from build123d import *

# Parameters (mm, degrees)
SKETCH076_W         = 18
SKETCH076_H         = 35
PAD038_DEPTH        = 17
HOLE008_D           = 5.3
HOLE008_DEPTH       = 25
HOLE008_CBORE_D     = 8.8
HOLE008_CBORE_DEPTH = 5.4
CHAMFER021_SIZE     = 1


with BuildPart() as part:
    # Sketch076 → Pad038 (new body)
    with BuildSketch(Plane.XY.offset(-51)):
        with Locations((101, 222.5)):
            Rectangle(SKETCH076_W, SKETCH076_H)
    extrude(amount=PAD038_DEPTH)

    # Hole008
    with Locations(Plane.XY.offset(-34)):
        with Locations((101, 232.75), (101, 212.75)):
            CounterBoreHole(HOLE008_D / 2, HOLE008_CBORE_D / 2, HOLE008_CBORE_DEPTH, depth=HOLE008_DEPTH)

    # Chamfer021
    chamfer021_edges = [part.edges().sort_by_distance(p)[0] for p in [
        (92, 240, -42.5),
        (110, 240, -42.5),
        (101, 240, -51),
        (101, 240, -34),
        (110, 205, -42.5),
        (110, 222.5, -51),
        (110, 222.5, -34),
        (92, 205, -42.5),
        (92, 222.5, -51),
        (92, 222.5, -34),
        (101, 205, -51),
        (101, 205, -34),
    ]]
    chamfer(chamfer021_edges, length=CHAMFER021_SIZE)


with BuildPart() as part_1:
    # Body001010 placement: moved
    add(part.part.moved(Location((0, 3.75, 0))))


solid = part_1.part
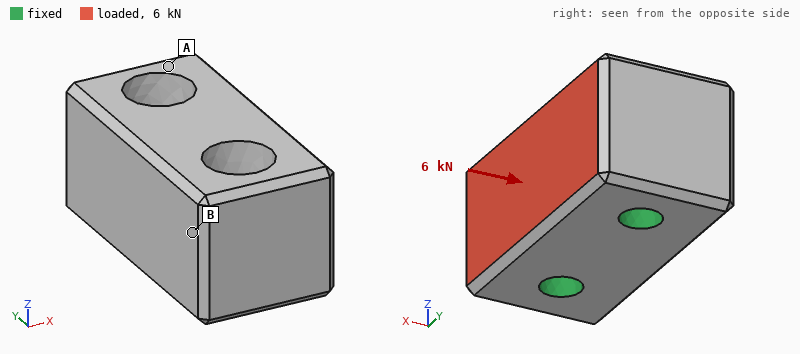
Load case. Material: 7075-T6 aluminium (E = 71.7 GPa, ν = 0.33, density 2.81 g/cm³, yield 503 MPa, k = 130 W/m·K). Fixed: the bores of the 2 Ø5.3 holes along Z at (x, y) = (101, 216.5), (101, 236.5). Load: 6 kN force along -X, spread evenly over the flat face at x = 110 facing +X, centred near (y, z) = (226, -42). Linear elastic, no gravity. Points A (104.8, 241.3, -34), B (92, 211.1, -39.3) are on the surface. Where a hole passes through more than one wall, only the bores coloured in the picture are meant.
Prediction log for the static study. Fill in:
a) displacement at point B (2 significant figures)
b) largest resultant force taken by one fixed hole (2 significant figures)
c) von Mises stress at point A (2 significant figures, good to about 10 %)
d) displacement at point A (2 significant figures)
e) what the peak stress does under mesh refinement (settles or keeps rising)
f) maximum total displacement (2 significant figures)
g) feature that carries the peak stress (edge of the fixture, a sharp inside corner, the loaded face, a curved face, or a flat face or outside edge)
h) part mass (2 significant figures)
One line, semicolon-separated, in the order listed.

1.9 µm; 3.1 kN; 12 MPa; 3.6 µm; keeps rising; 5.3 µm; edge of the fixture; 26 g
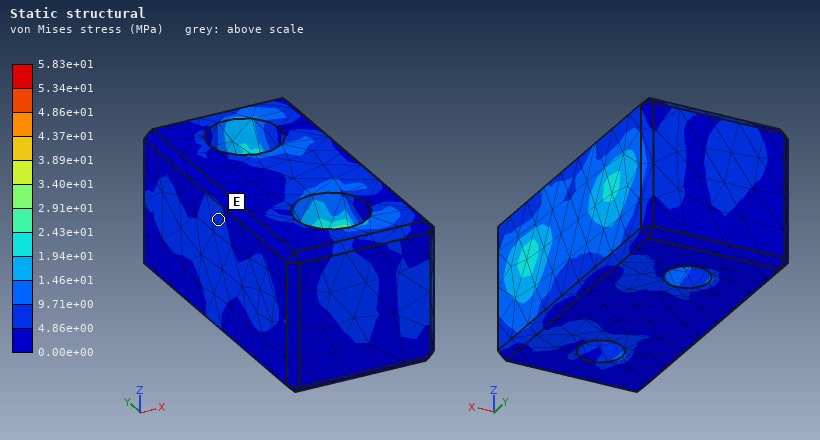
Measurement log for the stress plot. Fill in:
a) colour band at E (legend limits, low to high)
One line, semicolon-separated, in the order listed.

4.86e+00 to 9.71e+00 MPa
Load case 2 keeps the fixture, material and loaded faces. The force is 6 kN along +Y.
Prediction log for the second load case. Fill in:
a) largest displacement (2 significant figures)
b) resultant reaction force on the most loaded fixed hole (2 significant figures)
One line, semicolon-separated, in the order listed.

8.2 µm; 3.7 kN
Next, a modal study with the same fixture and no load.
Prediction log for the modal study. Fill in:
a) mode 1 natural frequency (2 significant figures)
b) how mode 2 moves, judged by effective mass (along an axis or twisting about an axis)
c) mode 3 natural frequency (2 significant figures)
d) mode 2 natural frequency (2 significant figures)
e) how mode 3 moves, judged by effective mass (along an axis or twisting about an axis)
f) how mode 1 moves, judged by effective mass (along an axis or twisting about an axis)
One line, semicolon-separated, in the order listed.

39 kHz; twisting about Z; 55 kHz; 51 kHz; along Y; along X
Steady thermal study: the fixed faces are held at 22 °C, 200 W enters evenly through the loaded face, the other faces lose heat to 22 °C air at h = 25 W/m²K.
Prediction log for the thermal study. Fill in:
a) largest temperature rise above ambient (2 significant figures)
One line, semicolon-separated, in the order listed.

33 K
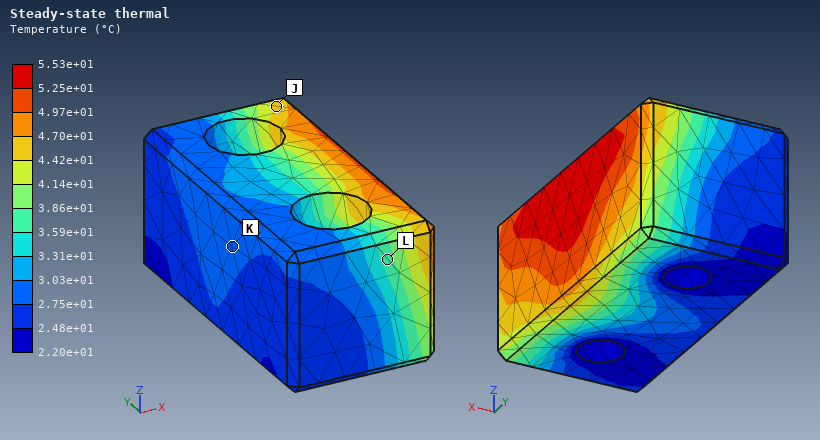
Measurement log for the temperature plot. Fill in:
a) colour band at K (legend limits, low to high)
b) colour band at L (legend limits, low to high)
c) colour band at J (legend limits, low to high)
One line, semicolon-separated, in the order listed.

2.75e+01 to 3.03e+01 °C; 3.59e+01 to 3.86e+01 °C; 4.42e+01 to 4.70e+01 °C
